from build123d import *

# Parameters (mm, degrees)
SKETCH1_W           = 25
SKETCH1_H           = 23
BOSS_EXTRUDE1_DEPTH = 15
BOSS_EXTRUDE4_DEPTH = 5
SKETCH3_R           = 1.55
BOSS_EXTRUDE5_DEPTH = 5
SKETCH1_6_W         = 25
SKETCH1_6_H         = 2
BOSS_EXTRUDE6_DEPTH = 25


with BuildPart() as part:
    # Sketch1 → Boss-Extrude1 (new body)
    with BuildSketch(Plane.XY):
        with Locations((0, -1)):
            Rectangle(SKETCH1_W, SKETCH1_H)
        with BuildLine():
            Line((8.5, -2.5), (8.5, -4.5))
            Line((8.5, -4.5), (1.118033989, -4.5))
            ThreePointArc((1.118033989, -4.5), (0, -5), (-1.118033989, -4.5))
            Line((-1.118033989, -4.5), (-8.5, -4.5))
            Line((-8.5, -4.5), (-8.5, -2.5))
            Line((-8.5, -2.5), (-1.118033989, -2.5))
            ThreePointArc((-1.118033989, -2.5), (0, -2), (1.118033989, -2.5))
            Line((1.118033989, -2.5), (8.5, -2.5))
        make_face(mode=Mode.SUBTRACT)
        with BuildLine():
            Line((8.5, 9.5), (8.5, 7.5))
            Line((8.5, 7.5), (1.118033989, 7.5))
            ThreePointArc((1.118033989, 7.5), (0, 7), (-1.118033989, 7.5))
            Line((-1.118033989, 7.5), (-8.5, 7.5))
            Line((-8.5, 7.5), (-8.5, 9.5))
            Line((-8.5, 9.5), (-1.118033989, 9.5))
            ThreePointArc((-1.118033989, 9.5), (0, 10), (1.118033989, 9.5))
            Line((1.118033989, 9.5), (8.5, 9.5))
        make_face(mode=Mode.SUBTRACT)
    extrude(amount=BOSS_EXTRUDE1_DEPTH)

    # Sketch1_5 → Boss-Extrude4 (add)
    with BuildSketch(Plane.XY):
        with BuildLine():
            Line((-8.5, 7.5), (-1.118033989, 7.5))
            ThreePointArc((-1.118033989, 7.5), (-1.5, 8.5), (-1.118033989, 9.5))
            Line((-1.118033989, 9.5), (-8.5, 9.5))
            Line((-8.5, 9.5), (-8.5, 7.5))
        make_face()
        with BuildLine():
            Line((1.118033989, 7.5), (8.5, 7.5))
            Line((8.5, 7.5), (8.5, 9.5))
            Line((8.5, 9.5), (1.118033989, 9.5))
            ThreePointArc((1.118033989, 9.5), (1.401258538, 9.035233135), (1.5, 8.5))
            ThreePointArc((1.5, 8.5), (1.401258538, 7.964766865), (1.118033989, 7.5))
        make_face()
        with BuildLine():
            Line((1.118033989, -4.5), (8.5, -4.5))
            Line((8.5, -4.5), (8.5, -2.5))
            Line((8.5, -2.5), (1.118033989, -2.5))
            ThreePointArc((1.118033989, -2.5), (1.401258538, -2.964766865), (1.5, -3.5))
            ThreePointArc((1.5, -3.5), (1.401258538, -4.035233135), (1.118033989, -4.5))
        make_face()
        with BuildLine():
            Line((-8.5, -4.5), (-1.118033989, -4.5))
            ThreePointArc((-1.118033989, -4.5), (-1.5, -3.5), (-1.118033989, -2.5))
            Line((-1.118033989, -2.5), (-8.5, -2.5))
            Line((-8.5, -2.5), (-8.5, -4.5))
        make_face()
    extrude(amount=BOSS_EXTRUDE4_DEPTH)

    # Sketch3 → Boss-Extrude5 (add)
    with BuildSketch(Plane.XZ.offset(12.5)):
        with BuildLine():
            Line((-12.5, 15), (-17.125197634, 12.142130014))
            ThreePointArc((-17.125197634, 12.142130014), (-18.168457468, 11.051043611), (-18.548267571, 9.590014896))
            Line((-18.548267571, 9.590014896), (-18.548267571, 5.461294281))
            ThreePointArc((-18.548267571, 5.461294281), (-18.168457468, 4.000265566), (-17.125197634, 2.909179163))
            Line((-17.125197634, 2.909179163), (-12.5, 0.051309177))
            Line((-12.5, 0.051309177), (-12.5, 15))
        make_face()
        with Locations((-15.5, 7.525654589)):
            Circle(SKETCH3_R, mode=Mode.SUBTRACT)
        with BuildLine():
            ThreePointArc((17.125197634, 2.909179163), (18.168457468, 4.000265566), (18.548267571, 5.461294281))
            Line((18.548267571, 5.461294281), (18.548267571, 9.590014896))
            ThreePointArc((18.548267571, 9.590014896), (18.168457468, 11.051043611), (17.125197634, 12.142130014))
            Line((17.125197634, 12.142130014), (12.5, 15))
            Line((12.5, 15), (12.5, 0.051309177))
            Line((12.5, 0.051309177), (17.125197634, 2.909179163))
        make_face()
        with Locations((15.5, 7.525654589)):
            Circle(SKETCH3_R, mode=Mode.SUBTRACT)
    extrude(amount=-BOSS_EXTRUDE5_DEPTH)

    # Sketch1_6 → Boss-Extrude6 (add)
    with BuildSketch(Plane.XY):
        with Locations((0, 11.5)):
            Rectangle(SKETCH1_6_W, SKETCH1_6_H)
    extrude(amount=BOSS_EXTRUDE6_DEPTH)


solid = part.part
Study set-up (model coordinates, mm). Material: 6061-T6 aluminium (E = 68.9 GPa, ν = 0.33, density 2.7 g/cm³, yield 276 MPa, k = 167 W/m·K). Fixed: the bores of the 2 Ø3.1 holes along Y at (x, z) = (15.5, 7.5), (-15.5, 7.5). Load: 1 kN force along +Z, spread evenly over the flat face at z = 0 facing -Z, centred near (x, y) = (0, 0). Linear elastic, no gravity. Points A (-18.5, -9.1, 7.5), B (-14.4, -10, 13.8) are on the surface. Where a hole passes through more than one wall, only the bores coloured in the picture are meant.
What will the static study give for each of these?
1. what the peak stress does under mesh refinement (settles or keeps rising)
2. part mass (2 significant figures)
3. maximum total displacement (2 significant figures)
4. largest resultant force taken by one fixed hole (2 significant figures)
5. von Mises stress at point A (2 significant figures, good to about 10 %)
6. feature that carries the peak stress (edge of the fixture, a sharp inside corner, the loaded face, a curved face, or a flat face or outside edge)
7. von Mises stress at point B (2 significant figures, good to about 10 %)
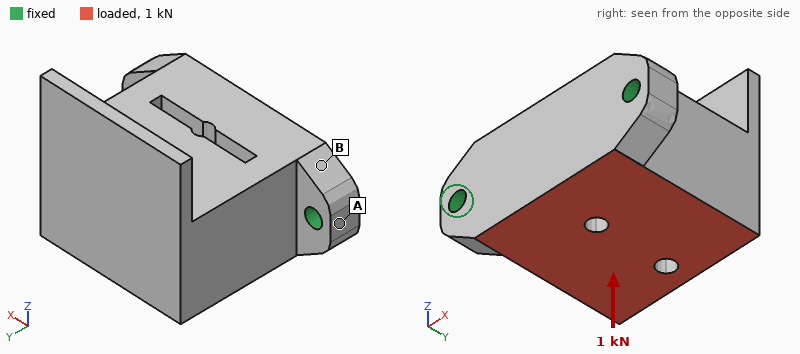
keeps rising
26 g
64 µm
500 N
24 MPa
edge of the fixture
53 MPa
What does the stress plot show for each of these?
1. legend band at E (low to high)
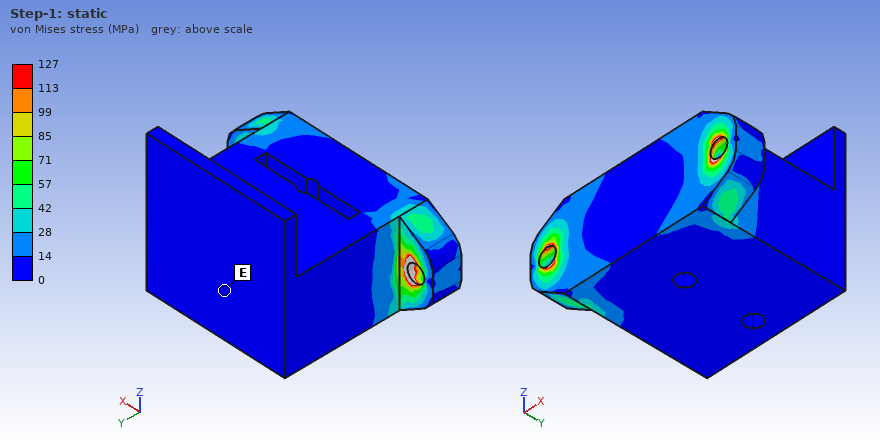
0 to 14 MPa
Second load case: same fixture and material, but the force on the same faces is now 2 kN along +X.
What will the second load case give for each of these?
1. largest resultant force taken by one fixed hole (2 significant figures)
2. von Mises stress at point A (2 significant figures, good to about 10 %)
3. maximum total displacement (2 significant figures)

1.3 kN
12 MPa
16 µm
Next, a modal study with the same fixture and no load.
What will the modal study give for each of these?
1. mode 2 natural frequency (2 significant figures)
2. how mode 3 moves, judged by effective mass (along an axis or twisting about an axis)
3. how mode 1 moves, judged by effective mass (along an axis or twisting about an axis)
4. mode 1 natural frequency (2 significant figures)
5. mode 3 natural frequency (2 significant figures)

11 kHz
along X
along Z
4900 Hz
13 kHz
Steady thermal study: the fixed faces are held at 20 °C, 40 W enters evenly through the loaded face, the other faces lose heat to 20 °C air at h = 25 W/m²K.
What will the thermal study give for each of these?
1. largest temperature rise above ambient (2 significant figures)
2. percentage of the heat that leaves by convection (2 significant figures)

21 K
3.4 %
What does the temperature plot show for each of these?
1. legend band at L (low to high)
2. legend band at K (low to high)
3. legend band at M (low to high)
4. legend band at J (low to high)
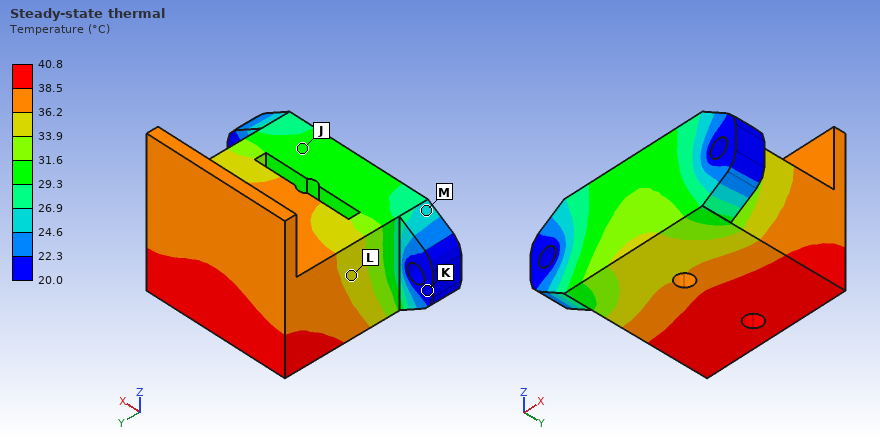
33.9 to 36.2 °C
20.0 to 22.3 °C
24.6 to 26.9 °C
29.3 to 31.6 °C
